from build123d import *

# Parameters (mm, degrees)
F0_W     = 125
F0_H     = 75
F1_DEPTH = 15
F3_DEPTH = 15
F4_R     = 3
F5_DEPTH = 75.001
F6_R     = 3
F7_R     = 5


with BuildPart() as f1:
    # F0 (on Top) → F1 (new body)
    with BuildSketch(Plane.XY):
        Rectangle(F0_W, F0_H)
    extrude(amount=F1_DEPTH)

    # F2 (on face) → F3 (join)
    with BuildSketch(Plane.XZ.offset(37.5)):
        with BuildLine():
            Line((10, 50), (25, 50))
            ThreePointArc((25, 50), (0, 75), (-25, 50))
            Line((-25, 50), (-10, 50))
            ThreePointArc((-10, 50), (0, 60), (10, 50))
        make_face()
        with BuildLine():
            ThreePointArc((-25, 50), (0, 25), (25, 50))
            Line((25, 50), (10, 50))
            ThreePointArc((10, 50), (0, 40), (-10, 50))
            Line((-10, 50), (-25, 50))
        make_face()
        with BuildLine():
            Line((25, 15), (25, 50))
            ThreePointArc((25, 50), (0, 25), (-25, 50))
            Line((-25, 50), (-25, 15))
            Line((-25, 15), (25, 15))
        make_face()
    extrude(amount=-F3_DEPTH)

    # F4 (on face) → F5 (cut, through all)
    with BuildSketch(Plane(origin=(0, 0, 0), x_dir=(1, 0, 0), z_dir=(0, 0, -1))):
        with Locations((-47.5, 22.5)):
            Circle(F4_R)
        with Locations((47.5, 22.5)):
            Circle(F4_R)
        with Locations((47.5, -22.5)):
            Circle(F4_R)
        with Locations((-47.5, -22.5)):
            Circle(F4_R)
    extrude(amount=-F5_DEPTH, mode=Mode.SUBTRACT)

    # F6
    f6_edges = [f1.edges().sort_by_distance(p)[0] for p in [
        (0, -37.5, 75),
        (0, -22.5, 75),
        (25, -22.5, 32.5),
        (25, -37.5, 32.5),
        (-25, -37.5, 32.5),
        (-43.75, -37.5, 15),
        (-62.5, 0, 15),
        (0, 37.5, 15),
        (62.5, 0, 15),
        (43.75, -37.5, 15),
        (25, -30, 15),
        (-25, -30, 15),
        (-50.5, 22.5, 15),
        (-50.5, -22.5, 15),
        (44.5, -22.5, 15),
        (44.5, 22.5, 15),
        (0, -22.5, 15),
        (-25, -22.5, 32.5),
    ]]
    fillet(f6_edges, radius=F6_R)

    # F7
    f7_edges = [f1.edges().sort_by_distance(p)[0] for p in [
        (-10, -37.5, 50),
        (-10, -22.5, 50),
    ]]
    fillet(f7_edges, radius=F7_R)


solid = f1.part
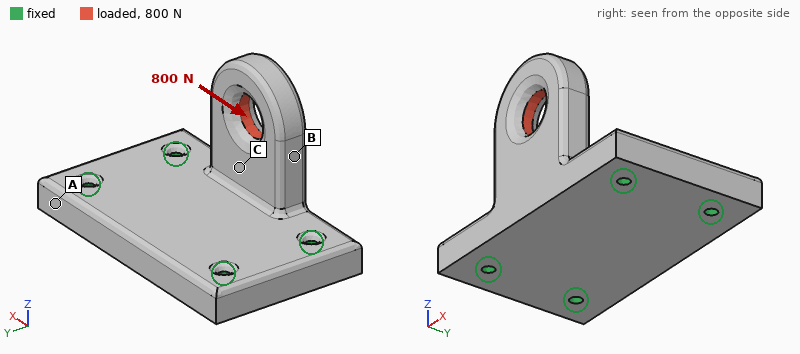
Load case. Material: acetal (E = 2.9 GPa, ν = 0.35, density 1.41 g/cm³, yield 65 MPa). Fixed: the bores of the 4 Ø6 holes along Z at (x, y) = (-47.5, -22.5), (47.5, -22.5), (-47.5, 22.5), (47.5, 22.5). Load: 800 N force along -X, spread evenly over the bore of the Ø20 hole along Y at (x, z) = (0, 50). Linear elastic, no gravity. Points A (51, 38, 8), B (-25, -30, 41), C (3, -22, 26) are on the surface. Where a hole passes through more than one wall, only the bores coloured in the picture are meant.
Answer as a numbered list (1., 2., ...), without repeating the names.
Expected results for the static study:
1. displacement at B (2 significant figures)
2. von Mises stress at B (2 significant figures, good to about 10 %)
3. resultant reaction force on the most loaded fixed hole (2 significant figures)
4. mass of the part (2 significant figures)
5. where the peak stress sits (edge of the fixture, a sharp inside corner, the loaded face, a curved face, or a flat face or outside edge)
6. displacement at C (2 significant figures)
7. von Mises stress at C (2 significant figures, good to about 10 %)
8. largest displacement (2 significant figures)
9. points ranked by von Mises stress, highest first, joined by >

1. 0.17 mm
2. 2.5 MPa
3. 550 N
4. 240 g
5. a curved face
6. 0.072 mm
7. 3.7 MPa
8. 0.30 mm
9. C > B > A
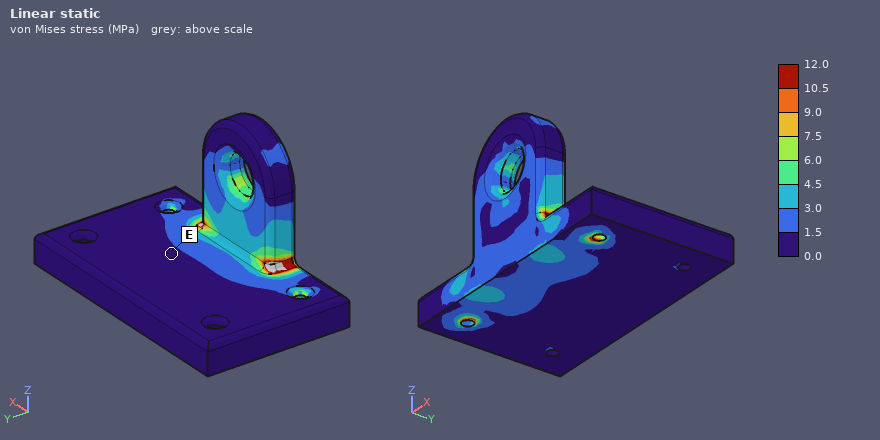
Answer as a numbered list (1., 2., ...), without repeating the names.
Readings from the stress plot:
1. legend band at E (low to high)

1. 0.0 to 1.5 MPa
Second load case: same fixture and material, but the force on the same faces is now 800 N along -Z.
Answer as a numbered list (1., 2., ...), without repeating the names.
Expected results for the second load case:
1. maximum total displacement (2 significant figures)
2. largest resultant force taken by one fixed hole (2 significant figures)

1. 0.23 mm
2. 460 N
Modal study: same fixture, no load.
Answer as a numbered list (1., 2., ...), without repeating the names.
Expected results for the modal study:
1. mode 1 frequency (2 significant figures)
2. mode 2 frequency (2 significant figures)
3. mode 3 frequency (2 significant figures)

1. 740 Hz
2. 1500 Hz
3. 1600 Hz
